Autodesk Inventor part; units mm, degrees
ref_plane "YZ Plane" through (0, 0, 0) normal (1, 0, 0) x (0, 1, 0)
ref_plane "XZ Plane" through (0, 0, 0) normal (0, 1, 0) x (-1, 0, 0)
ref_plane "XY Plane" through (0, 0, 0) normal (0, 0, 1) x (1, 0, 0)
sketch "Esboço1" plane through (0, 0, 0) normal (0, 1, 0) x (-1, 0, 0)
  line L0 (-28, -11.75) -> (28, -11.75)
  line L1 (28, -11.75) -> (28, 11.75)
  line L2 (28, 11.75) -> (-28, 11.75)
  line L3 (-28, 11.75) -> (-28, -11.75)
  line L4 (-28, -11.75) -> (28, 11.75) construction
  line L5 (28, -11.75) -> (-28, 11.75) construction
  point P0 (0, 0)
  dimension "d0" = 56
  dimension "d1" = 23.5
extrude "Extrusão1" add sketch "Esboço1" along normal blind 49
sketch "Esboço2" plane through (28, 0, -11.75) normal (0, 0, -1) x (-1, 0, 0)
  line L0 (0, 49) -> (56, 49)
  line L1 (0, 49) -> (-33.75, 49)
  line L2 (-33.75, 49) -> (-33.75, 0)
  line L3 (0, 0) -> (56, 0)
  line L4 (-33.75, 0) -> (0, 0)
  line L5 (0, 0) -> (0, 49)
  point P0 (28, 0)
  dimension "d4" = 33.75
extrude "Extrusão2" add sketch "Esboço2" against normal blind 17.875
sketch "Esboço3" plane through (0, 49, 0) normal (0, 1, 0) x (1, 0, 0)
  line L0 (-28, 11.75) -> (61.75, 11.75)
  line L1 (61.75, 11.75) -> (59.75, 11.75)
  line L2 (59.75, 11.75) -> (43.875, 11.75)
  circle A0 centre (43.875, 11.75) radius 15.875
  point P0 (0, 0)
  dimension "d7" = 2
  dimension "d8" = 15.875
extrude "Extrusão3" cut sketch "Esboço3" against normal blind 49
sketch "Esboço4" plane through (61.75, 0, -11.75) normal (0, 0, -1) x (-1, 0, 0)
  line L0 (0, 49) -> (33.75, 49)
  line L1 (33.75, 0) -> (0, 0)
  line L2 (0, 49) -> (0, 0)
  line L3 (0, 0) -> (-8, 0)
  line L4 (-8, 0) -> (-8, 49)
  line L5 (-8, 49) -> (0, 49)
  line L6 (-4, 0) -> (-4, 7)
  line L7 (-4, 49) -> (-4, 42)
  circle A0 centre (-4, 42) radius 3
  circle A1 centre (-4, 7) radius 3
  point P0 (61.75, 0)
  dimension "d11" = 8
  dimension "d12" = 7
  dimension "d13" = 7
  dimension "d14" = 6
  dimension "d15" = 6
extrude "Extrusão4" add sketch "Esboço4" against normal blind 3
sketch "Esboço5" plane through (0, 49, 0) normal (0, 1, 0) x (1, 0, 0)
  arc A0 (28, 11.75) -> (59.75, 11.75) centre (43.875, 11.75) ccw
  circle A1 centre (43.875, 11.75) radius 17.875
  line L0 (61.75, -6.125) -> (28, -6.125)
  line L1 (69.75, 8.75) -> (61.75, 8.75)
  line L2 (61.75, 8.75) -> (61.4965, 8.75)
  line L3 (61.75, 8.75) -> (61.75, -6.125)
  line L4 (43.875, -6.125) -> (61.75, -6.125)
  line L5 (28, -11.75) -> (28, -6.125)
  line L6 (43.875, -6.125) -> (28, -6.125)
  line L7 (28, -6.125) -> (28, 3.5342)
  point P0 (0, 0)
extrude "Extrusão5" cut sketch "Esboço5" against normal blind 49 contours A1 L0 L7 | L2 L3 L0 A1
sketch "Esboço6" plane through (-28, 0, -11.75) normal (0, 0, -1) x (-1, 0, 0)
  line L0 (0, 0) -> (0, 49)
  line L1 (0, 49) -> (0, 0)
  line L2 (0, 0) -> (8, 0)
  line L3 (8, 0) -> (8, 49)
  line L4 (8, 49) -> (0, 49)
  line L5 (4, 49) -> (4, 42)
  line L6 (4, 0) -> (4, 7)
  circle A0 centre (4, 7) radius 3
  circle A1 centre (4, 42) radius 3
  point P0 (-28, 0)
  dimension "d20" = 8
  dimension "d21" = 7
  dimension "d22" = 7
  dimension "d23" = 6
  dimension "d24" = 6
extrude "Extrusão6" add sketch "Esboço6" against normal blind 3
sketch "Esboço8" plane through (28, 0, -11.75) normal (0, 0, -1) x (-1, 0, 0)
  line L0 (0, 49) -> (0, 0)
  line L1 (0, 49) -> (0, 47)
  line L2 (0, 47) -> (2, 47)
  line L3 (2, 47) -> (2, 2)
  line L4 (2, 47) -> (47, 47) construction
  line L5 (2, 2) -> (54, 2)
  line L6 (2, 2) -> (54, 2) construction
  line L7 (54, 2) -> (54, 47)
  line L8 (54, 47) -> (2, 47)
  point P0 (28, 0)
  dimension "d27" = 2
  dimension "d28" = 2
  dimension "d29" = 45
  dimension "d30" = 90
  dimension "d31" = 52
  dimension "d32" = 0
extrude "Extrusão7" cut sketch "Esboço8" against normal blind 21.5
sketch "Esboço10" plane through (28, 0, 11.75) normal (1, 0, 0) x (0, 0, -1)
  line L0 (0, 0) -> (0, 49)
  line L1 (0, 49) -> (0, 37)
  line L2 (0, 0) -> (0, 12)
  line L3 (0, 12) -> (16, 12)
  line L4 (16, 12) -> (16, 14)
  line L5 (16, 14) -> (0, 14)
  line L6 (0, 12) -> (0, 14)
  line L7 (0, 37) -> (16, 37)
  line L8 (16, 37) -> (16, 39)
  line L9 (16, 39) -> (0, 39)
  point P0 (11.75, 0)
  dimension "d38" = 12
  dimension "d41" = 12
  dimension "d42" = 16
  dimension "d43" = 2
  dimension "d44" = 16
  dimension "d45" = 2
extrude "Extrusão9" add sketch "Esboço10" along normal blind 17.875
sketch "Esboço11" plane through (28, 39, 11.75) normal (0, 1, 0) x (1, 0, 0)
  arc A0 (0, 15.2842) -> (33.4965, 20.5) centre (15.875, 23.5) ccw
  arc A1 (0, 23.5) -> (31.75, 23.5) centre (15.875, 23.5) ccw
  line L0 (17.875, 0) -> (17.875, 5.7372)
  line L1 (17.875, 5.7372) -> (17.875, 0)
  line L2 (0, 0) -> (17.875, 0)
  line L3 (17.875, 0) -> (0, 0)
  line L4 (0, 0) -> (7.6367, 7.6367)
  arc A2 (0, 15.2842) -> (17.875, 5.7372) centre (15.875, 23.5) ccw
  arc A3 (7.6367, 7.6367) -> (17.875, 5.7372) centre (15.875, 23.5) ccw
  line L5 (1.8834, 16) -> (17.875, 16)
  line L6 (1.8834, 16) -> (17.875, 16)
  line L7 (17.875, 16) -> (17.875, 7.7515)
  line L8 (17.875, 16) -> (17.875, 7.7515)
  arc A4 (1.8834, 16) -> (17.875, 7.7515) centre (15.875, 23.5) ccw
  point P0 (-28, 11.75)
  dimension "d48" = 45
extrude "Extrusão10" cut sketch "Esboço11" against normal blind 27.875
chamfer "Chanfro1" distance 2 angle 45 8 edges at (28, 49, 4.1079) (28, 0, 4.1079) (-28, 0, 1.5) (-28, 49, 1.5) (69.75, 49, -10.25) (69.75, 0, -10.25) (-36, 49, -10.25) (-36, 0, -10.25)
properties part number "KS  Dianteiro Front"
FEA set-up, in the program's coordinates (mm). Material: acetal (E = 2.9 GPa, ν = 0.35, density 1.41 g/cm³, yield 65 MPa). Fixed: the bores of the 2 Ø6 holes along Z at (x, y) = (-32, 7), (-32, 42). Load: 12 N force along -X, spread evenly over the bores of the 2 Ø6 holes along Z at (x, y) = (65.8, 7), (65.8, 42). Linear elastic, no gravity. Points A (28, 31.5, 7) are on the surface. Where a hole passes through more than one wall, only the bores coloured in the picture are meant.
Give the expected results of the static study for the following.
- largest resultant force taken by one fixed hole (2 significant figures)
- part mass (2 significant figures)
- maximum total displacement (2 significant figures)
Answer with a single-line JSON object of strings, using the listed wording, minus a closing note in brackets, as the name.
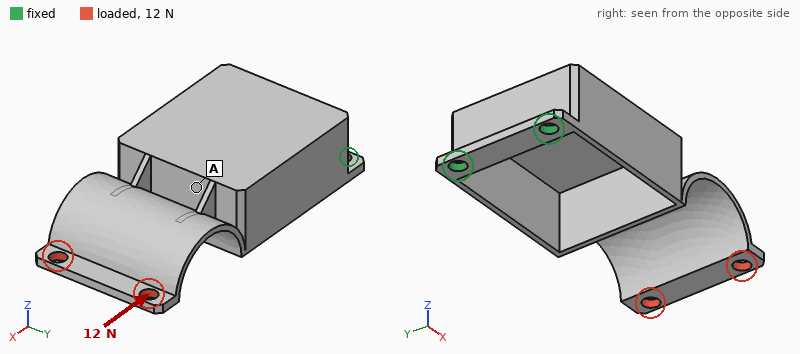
{"largest resultant force taken by one fixed hole": "6.0 N", "part mass": "29 g", "maximum total displacement": "1.3 mm"}
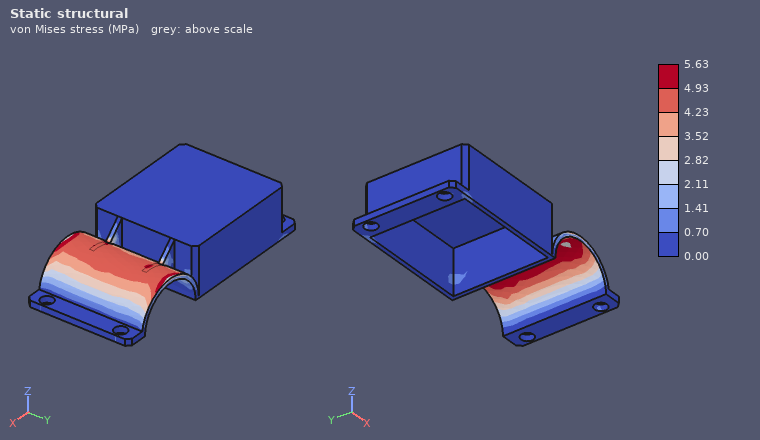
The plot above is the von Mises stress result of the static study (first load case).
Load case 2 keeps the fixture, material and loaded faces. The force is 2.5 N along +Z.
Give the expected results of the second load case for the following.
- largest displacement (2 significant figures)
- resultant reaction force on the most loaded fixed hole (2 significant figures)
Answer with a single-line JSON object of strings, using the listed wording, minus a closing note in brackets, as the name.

{"largest displacement": "1.3 mm", "resultant reaction force on the most loaded fixed hole": "2.9 N"}
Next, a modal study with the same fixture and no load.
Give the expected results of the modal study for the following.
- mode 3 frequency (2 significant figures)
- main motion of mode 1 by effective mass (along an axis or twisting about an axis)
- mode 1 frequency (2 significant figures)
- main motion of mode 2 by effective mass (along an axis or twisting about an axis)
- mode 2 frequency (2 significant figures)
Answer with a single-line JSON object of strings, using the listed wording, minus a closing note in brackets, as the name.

{"mode 3 frequency": "300 Hz", "main motion of mode 1 by effective mass": "along Z", "mode 1 frequency": "89 Hz", "main motion of mode 2 by effective mass": "along Y", "mode 2 frequency": "130 Hz"}
